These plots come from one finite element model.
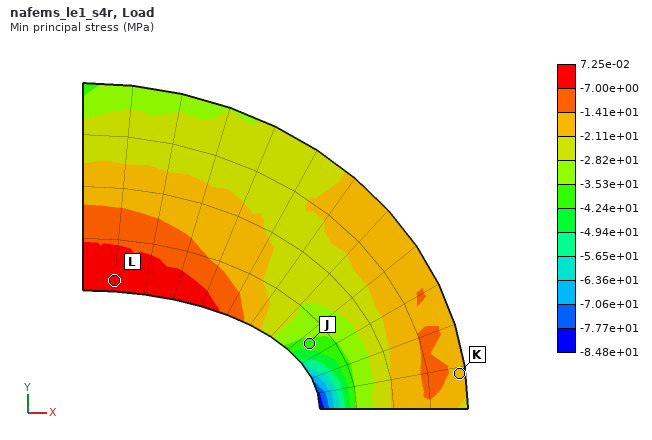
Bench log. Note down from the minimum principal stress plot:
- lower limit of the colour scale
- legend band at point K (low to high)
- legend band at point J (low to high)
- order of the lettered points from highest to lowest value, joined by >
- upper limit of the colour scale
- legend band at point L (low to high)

-8.48e+01 MPa
-2.11e+01 to -1.41e+01 MPa
-4.24e+01 to -3.53e+01 MPa
L > K > J
7.25e-02 MPa
-7.00e+00 to 7.25e-02 MPa
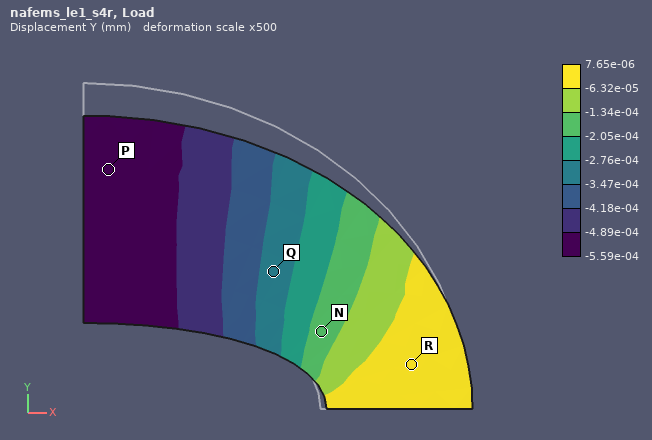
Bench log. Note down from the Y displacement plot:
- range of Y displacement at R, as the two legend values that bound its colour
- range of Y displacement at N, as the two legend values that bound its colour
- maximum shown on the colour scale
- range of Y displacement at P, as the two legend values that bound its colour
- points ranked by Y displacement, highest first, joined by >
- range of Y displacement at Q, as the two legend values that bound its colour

-6.32e-05 to 7.65e-06 mm
-2.05e-04 to -1.34e-04 mm
7.65e-06 mm
-5.59e-04 to -4.89e-04 mm
R > N > Q > P
-3.47e-04 to -2.76e-04 mm
